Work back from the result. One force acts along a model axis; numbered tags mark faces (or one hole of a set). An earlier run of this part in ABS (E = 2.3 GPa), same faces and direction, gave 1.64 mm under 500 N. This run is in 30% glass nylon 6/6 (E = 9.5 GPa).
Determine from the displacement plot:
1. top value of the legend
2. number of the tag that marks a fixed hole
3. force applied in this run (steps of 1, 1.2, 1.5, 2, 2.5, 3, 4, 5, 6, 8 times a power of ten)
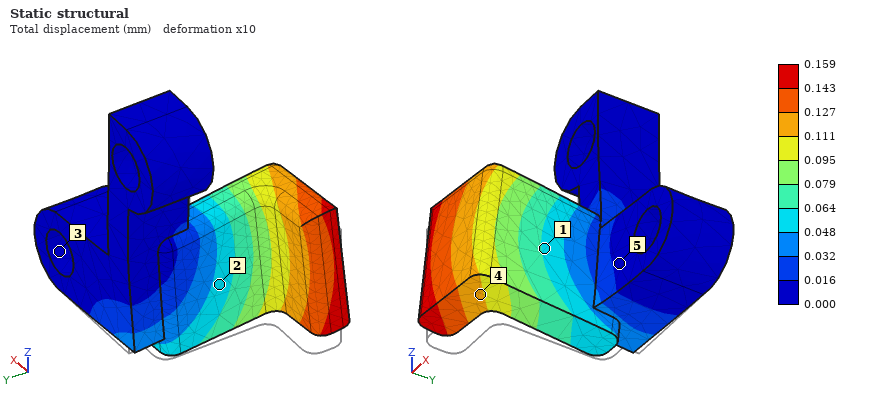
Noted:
0.159 mm
3
200 N
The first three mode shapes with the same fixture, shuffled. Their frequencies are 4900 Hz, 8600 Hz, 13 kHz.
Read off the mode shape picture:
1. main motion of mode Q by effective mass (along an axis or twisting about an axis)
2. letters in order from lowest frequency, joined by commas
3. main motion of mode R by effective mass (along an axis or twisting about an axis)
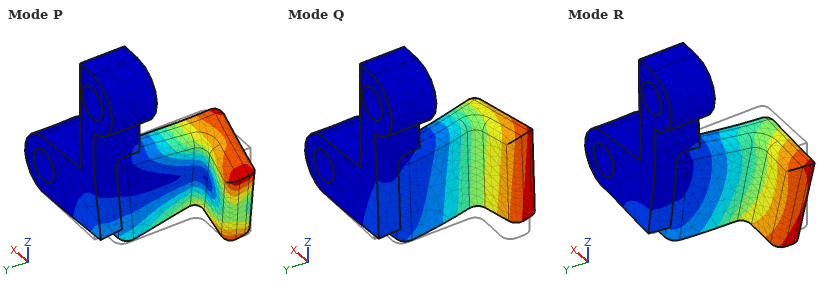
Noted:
along X
Q, R, P
along Z
